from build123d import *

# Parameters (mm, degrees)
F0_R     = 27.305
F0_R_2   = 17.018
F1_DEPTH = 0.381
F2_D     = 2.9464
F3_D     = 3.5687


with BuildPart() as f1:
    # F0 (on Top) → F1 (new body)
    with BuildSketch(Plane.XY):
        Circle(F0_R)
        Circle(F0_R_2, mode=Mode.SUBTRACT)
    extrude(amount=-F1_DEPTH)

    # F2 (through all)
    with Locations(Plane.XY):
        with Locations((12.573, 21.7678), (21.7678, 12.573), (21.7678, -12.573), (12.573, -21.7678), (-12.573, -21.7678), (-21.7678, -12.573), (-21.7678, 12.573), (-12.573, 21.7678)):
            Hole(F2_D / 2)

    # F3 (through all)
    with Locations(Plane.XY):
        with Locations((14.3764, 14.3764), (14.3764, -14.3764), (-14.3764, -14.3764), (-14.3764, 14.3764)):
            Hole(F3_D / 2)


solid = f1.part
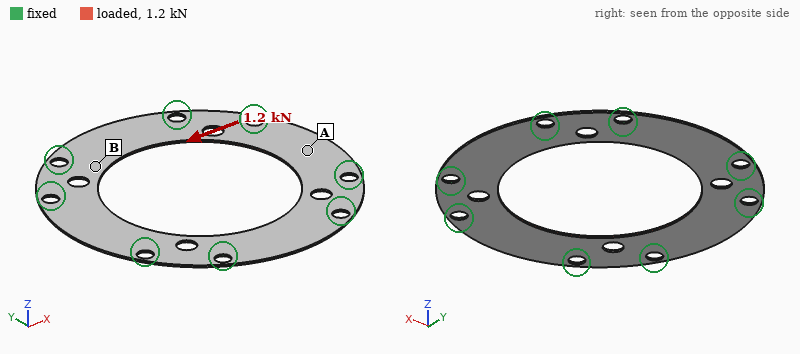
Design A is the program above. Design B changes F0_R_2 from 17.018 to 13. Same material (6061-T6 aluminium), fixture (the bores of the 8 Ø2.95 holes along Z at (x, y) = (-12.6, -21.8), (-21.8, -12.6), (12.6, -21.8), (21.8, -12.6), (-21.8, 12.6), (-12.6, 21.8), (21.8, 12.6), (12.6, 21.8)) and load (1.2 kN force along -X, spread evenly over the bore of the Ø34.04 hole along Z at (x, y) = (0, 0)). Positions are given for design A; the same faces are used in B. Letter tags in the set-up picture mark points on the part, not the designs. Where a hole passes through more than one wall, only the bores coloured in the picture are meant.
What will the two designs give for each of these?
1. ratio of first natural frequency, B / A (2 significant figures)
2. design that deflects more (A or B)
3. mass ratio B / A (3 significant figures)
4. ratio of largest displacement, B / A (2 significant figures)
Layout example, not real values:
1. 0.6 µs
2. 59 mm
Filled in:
1. 0.69
2. A
3. 1.28
4. 0.87
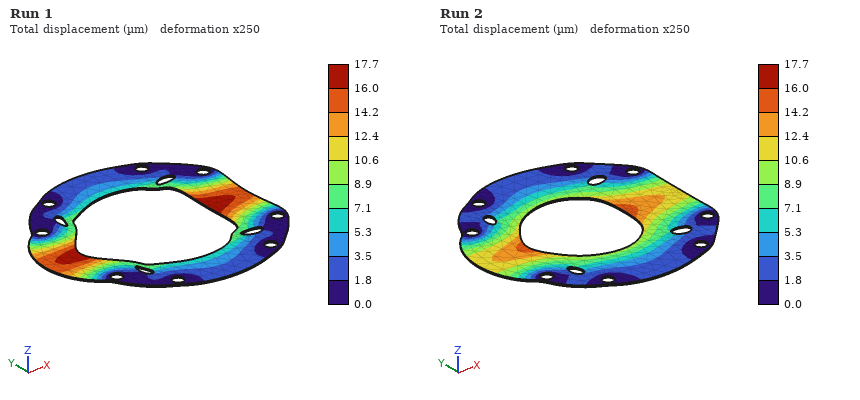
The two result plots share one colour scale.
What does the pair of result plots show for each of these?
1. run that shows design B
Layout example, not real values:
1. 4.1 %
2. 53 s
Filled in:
1. Run 2
